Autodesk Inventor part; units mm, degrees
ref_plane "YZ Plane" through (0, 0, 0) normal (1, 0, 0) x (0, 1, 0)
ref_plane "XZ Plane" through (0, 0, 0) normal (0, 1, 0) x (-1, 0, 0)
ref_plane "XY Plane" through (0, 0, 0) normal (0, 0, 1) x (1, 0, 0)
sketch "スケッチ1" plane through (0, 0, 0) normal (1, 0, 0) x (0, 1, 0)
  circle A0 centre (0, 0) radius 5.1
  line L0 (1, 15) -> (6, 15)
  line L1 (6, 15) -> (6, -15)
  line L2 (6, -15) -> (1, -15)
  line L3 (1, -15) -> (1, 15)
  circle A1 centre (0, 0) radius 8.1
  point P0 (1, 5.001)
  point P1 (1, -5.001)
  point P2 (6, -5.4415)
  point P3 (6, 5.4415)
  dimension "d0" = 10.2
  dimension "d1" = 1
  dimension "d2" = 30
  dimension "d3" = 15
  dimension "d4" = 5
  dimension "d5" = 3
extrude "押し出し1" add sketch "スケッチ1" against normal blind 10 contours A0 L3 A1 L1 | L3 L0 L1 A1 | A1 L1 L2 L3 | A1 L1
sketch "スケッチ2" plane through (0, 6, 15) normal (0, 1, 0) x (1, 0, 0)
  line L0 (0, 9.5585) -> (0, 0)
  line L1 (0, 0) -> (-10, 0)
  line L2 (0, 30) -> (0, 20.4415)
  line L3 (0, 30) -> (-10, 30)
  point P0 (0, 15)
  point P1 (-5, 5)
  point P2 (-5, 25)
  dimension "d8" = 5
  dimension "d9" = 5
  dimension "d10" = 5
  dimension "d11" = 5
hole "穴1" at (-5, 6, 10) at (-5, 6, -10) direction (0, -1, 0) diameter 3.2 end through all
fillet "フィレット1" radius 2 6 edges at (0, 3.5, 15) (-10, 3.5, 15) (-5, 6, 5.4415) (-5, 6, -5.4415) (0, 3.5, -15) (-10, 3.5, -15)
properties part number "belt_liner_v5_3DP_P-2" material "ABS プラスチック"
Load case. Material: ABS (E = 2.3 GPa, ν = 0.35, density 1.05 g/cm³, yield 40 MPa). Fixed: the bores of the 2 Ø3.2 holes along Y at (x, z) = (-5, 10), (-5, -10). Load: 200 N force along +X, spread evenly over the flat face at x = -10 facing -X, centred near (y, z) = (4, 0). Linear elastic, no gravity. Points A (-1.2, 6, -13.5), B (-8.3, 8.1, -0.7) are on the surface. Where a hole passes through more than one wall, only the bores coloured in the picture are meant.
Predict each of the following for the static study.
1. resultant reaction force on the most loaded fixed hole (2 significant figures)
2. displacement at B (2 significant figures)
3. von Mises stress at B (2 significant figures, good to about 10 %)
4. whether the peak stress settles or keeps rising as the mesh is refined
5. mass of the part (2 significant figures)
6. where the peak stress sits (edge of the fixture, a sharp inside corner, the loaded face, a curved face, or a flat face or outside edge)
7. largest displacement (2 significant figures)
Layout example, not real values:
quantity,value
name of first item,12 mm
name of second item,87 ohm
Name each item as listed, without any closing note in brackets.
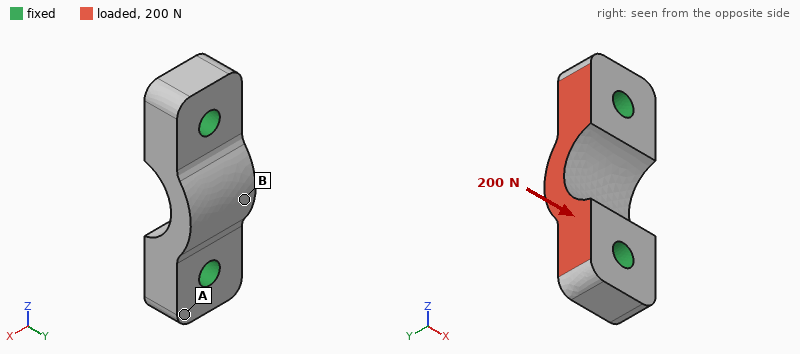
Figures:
quantity,value
resultant reaction force on the most loaded fixed hole,100 N
displacement at B,30 µm
von Mises stress at B,1.8 MPa
whether the peak stress settles or keeps rising as the mesh is refined,keeps rising
mass of the part,1.3 g
where the peak stress sits,edge of the fixture
largest displacement,34 µm
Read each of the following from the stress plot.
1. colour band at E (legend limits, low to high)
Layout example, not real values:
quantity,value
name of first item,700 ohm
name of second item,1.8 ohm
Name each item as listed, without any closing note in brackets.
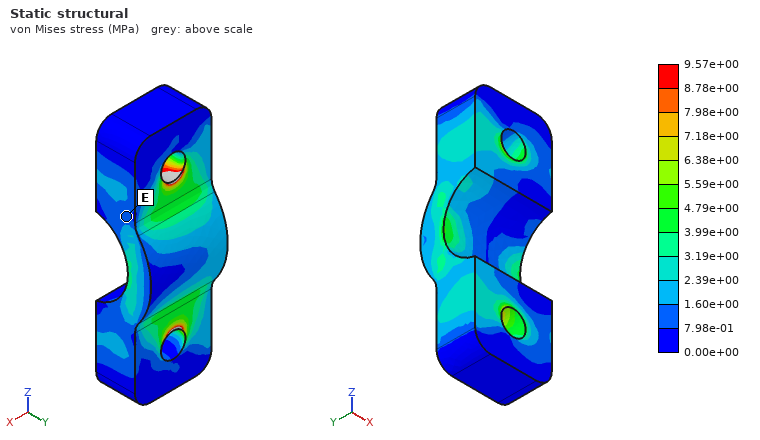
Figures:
quantity,value
colour band at E,7.98e-01 to 1.60e+00 MPa
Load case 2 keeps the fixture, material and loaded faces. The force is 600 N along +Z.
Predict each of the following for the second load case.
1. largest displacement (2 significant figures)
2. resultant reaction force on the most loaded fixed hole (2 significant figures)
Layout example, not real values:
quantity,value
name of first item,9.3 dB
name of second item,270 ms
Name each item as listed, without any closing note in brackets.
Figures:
quantity,value
largest displacement,57 µm
resultant reaction force on the most loaded fixed hole,310 N
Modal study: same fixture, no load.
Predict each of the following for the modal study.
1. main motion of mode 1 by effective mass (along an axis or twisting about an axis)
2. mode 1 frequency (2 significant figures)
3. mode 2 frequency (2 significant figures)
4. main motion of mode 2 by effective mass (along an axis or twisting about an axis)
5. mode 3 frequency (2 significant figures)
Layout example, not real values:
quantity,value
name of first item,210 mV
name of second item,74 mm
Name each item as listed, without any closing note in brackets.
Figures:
quantity,value
main motion of mode 1 by effective mass,along X
mode 1 frequency,14 kHz
mode 2 frequency,18 kHz
main motion of mode 2 by effective mass,along Y
mode 3 frequency,23 kHz
